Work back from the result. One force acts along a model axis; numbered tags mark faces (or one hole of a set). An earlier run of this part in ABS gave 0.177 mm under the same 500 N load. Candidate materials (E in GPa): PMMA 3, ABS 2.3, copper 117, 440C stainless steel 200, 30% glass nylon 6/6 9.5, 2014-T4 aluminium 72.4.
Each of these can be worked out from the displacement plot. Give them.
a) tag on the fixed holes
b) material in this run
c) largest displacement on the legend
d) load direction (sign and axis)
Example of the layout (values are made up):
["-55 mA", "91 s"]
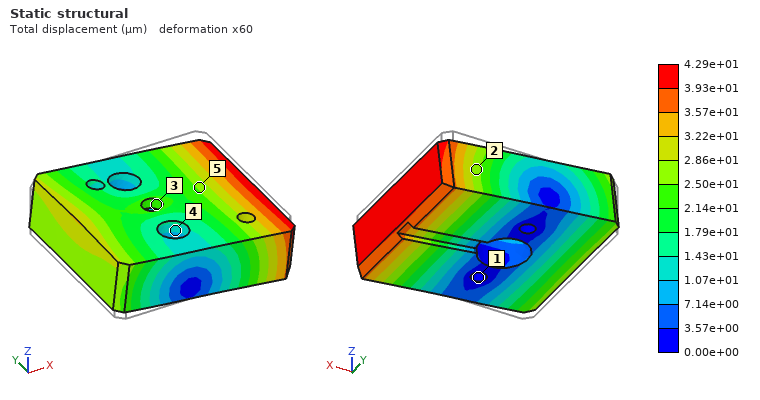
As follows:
["1", "30% glass nylon 6/6", "4.29e+01 µm", "+X"]
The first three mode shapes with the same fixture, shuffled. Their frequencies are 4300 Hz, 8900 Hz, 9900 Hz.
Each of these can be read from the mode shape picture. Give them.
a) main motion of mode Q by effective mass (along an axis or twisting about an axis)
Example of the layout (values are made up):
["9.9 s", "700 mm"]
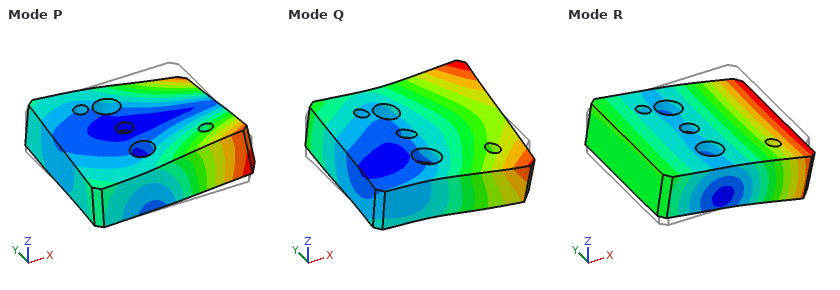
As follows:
["along Y"]
